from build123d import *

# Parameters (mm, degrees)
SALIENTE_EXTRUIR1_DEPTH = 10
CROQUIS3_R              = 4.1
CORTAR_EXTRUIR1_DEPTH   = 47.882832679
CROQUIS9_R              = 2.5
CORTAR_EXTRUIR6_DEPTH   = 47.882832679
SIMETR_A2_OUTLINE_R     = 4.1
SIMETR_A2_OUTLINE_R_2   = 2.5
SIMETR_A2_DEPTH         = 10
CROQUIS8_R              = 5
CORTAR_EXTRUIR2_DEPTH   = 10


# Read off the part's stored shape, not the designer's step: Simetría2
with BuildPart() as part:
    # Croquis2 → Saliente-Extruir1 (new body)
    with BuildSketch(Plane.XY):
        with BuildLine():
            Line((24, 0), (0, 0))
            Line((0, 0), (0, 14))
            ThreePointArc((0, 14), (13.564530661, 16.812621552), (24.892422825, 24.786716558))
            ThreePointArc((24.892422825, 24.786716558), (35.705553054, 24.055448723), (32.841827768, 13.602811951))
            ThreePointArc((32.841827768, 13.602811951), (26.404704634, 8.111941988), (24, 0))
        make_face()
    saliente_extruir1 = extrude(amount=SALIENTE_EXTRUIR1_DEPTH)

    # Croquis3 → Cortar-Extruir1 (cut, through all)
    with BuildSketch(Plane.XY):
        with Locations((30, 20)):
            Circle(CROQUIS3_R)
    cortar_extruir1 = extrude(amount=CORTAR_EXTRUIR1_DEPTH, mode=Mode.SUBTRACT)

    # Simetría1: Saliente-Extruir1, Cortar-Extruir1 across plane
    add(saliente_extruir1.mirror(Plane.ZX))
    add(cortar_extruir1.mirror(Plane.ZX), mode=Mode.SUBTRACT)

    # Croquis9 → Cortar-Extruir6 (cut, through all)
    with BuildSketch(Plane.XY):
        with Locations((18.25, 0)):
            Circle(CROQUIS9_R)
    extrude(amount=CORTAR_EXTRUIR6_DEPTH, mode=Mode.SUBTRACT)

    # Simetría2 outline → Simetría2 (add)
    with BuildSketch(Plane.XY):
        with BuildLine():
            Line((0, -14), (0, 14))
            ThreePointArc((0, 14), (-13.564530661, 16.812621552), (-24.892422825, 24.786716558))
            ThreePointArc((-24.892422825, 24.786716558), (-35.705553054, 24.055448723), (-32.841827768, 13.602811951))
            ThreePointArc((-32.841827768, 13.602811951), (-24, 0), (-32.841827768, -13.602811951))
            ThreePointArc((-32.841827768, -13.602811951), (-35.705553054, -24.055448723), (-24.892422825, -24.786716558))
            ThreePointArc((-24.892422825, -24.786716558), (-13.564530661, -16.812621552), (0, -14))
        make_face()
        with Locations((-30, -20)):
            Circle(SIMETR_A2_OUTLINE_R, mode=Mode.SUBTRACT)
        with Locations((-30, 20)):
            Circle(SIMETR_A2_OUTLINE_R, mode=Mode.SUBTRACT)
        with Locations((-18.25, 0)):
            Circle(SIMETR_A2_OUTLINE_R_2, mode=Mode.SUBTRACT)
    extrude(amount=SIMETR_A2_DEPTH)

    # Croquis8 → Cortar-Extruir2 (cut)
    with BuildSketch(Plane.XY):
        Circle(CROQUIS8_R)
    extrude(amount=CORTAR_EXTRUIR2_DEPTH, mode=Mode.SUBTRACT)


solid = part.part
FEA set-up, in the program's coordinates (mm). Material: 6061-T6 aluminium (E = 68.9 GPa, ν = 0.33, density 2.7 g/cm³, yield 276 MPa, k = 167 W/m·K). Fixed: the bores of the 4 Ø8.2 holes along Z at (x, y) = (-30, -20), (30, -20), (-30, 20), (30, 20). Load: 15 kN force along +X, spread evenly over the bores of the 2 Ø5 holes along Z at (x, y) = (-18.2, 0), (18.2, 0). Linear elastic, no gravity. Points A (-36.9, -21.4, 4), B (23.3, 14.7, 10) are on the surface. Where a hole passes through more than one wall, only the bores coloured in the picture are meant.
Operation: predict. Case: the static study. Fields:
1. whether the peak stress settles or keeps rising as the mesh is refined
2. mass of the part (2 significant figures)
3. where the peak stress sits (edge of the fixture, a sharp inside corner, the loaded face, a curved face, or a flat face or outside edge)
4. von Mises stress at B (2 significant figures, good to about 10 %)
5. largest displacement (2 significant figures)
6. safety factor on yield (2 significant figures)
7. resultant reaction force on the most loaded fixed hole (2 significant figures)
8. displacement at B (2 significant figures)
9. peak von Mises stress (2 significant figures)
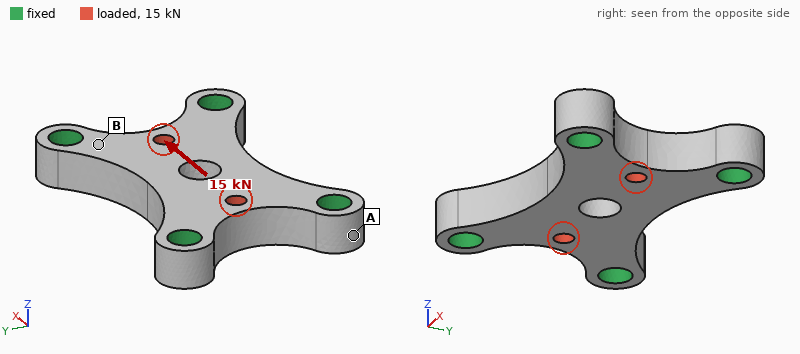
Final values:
settles
55 g
the loaded face
34 MPa
22 µm
2.5
4.5 kN
3.3 µm
110 MPa
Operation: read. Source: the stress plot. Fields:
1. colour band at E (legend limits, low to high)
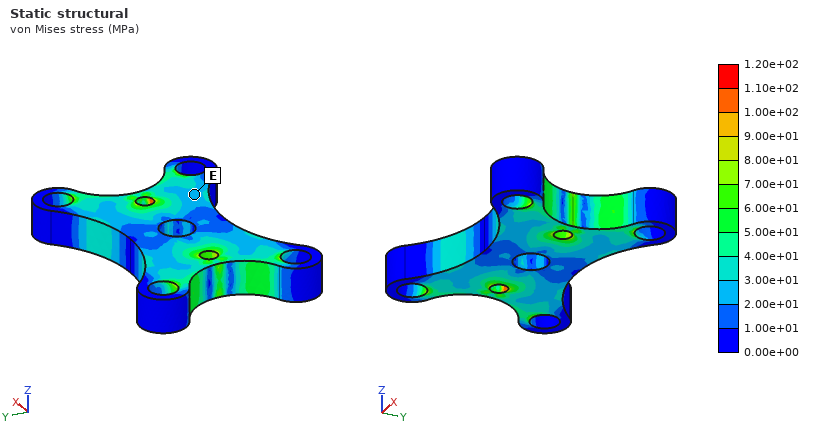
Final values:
2.00e+01 to 3.00e+01 MPa
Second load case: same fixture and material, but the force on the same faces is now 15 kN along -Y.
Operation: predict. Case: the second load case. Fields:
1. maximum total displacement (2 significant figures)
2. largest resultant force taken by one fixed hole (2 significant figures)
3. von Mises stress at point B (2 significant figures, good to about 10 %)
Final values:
15 µm
4.2 kN
41 MPa
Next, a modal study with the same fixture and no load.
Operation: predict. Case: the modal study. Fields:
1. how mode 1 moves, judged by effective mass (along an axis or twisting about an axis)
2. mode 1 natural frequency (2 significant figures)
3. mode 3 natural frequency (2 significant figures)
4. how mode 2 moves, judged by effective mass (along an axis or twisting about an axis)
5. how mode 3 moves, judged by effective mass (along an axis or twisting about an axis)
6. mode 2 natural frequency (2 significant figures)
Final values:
along Z
12 kHz
25 kHz
twisting about X
twisting about Y
22 kHz
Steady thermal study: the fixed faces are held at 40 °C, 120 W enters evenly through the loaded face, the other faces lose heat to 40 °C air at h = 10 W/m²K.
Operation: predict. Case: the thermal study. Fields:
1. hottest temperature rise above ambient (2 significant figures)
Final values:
26 K
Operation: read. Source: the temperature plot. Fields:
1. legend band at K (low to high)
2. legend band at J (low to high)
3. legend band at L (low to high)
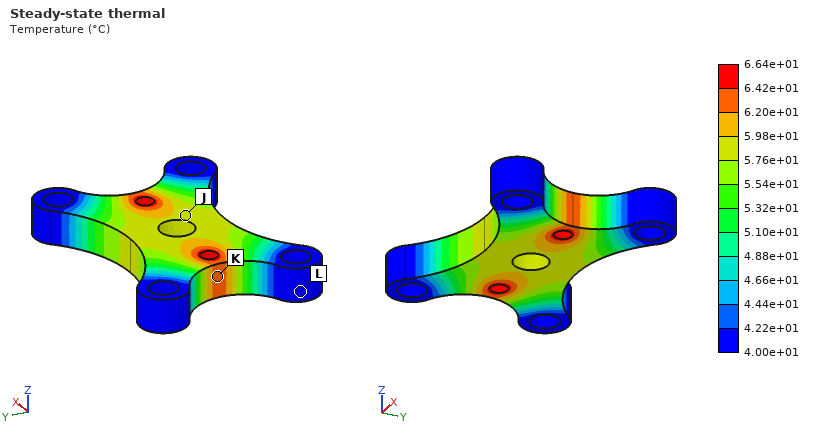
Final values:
6.20e+01 to 6.42e+01 °C
5.76e+01 to 5.98e+01 °C
4.00e+01 to 4.22e+01 °C
